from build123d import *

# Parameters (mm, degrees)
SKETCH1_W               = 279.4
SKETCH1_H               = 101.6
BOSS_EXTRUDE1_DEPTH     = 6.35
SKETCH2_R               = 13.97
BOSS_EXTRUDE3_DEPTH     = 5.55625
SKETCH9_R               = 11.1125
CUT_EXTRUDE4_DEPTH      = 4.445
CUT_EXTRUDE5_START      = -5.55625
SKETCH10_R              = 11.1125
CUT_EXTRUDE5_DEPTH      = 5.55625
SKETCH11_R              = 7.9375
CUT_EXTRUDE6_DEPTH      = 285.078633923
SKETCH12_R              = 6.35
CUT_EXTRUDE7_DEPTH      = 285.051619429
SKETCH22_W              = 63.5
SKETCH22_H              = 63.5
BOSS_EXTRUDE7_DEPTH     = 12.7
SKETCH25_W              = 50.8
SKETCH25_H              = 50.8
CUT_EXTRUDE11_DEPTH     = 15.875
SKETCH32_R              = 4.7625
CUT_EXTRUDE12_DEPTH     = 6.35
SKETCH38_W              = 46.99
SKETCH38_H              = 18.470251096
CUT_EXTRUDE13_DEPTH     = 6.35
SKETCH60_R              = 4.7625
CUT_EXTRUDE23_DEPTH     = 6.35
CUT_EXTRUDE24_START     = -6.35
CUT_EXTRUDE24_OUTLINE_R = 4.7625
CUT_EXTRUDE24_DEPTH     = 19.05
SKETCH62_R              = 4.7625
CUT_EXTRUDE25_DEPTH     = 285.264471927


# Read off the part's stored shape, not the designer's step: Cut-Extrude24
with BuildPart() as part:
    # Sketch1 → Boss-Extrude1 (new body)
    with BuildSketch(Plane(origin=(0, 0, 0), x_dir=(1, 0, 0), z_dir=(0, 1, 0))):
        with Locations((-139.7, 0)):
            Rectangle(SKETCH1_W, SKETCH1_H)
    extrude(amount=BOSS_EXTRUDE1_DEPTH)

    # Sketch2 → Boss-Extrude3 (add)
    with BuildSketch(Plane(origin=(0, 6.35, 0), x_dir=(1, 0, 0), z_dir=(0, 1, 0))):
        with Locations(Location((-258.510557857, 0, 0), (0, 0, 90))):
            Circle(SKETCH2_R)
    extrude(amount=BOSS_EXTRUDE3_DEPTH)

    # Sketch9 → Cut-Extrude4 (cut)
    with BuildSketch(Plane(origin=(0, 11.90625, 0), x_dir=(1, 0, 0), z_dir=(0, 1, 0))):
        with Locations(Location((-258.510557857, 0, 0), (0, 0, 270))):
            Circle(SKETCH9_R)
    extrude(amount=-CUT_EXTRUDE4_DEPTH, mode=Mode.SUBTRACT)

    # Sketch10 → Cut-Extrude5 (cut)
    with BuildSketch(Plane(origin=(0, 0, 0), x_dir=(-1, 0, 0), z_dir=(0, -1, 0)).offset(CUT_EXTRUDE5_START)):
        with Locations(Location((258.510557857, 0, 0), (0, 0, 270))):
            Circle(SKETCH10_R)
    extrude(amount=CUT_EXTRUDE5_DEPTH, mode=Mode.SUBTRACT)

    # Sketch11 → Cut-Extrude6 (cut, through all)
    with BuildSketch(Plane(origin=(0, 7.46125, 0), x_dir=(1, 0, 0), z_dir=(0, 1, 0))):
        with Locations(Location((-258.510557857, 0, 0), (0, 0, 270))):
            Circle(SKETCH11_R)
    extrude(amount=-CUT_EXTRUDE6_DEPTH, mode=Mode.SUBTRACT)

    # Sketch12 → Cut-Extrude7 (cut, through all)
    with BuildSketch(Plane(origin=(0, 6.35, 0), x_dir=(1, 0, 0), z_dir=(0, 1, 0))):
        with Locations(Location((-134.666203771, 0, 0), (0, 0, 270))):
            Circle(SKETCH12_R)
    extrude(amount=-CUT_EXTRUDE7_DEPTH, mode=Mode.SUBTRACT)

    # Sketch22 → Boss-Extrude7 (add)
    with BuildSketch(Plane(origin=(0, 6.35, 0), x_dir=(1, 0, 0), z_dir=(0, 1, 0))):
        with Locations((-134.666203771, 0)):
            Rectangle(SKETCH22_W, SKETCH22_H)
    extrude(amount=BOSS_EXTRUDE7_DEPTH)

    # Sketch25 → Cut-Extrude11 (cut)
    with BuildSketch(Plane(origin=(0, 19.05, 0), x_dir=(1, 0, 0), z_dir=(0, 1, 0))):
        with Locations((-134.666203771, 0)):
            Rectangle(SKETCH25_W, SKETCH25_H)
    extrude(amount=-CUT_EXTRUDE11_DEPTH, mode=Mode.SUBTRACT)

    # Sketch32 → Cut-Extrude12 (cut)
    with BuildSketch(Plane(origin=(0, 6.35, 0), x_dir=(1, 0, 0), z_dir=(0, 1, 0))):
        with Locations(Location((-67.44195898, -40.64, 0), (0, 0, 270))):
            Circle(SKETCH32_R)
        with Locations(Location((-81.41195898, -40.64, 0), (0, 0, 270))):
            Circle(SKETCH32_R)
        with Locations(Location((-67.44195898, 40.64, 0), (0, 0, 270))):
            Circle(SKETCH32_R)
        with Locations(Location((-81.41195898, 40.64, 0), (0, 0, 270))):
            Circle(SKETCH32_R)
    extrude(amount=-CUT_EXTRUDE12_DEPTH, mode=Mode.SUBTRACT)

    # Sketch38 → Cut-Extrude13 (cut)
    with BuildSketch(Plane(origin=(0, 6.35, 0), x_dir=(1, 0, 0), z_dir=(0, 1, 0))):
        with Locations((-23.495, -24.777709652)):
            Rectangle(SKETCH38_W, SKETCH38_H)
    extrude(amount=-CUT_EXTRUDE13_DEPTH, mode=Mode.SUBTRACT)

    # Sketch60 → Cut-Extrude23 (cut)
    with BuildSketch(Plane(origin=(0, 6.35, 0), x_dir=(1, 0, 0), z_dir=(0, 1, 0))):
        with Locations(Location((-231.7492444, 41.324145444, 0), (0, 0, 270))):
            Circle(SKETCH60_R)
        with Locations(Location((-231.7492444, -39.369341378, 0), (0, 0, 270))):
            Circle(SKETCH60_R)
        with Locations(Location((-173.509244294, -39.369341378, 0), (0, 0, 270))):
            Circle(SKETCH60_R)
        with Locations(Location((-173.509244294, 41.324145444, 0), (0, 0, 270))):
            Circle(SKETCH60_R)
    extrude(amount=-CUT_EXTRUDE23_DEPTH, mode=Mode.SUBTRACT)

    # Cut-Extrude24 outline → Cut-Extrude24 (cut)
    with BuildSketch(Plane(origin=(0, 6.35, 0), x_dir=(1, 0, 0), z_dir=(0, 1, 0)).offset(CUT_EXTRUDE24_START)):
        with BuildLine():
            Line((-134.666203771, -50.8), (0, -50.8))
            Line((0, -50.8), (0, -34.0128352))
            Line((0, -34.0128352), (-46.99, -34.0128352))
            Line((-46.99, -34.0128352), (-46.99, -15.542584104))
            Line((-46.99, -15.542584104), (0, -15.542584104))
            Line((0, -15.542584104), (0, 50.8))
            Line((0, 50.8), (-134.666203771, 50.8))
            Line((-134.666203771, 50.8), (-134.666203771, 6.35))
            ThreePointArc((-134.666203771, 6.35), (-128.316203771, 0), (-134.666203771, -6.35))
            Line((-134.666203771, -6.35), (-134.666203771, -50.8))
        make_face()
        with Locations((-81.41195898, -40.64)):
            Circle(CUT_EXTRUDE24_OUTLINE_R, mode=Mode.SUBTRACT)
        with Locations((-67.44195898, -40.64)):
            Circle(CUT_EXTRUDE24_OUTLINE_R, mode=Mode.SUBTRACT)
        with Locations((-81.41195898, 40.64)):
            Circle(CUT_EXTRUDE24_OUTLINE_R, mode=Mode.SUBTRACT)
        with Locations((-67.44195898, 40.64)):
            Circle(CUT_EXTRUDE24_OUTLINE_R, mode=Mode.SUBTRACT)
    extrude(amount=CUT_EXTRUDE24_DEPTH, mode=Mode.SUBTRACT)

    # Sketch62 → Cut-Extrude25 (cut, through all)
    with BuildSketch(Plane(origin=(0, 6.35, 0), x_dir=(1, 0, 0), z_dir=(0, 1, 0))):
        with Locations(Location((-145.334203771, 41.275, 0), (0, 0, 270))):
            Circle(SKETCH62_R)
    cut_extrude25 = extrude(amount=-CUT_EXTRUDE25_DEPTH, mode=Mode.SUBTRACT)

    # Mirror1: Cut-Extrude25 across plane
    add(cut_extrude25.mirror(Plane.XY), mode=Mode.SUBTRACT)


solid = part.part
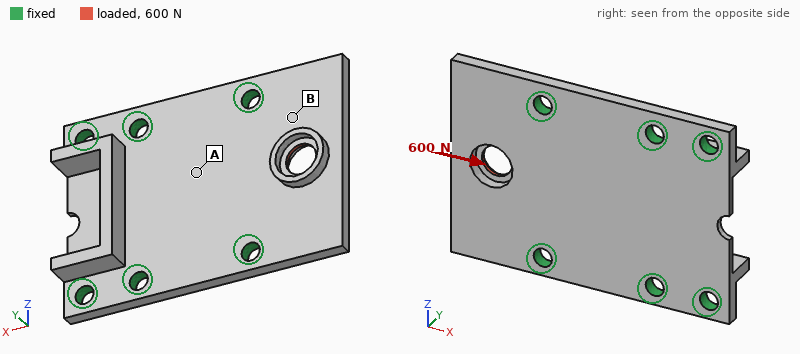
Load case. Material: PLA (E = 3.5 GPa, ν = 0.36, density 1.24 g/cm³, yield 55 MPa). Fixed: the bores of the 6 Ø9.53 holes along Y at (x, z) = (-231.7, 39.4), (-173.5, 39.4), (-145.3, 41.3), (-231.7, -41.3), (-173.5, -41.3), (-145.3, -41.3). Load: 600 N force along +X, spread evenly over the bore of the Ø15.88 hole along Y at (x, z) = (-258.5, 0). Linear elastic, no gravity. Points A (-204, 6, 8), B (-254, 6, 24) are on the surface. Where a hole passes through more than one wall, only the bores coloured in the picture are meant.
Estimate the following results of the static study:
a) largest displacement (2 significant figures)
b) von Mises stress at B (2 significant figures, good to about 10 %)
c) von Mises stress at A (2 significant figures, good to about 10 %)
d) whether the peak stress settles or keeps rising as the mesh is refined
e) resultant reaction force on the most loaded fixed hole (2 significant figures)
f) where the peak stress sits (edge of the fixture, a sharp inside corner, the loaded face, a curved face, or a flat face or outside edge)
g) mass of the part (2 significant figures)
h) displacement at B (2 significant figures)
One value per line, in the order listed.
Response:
0.30 mm
3.1 MPa
0.88 MPa
keeps rising
230 N
a sharp inside corner
120 g
0.079 mm
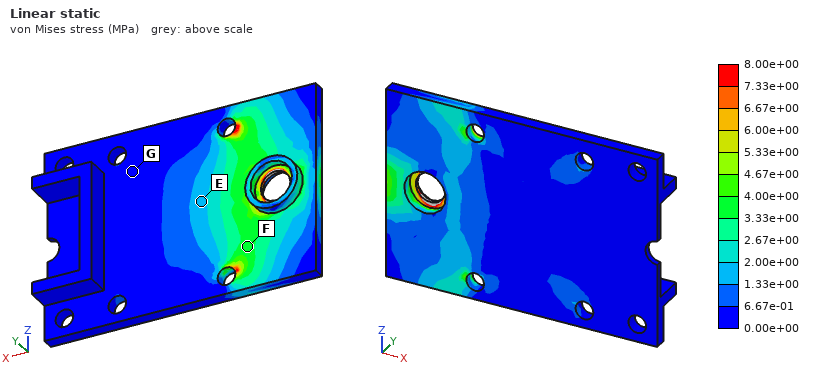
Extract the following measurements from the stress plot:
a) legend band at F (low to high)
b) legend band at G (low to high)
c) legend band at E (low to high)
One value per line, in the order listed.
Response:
3.33e+00 to 4.00e+00 MPa
0.00e+00 to 6.67e-01 MPa
1.33e+00 to 2.00e+00 MPa
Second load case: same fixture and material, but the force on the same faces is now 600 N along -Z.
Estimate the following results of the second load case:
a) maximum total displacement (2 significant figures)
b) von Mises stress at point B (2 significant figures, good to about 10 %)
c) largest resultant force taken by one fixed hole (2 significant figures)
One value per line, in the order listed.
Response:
84 µm
2.8 MPa
340 N
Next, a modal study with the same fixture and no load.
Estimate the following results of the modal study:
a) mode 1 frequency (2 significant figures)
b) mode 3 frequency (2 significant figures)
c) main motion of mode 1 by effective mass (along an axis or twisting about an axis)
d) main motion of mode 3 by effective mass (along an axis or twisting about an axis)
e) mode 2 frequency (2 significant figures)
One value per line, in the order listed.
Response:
700 Hz
1700 Hz
along Y
along Y
1200 Hz
